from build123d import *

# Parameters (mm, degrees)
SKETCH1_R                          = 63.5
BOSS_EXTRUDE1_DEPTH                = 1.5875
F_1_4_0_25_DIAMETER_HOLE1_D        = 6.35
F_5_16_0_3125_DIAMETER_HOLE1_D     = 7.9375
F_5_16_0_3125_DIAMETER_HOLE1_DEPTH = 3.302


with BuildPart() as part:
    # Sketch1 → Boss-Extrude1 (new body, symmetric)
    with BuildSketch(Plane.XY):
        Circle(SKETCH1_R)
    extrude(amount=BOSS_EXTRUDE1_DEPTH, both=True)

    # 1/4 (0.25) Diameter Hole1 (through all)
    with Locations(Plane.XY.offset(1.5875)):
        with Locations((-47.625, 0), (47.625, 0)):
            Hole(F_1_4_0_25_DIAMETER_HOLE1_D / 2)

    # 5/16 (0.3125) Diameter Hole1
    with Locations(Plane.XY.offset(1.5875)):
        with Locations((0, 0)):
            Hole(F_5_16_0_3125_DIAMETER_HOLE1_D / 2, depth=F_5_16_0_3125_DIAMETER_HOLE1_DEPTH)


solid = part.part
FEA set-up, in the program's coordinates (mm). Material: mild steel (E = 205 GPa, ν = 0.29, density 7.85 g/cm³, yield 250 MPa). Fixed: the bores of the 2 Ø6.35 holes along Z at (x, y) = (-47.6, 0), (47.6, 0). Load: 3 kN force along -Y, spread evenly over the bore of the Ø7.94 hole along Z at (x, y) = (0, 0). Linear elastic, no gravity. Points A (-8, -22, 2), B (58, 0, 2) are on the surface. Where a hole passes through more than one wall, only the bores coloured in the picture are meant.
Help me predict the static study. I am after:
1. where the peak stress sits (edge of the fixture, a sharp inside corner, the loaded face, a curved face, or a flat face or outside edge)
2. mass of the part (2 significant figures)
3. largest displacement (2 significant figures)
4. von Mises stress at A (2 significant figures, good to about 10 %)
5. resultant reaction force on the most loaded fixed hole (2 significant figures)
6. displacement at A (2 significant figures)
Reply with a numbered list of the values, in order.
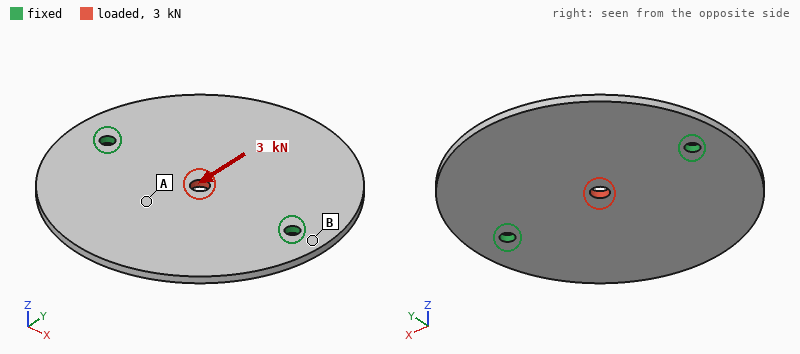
1. the loaded face
2. 310 g
3. 5.8 µm
4. 12 MPa
5. 1.5 kN
6. 3.7 µm
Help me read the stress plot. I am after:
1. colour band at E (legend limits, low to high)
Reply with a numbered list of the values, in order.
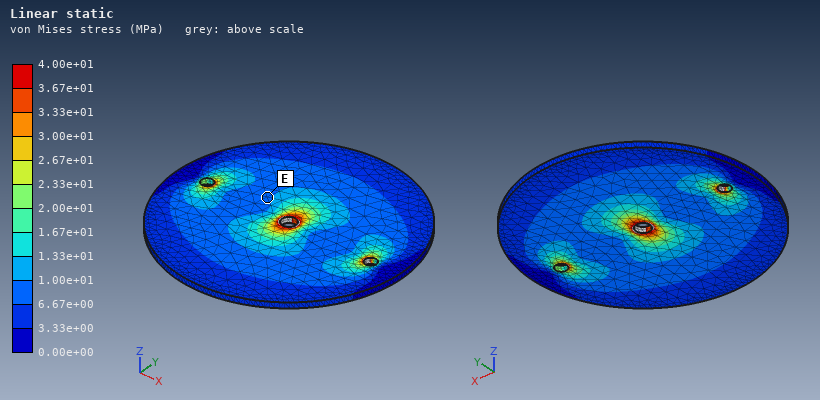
1. 6.67e+00 to 1.00e+01 MPa
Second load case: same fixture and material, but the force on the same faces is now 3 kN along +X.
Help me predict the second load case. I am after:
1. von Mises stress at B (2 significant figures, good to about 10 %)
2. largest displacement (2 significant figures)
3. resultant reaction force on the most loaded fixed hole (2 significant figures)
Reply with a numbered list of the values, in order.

1. 7.2 MPa
2. 4.4 µm
3. 1.5 kN
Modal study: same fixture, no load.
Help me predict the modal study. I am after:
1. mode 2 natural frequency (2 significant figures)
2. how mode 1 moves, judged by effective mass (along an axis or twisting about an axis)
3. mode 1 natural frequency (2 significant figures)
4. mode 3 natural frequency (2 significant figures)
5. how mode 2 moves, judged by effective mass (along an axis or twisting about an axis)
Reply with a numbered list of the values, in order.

1. 780 Hz
2. twisting about X
3. 600 Hz
4. 1700 Hz
5. along Z
